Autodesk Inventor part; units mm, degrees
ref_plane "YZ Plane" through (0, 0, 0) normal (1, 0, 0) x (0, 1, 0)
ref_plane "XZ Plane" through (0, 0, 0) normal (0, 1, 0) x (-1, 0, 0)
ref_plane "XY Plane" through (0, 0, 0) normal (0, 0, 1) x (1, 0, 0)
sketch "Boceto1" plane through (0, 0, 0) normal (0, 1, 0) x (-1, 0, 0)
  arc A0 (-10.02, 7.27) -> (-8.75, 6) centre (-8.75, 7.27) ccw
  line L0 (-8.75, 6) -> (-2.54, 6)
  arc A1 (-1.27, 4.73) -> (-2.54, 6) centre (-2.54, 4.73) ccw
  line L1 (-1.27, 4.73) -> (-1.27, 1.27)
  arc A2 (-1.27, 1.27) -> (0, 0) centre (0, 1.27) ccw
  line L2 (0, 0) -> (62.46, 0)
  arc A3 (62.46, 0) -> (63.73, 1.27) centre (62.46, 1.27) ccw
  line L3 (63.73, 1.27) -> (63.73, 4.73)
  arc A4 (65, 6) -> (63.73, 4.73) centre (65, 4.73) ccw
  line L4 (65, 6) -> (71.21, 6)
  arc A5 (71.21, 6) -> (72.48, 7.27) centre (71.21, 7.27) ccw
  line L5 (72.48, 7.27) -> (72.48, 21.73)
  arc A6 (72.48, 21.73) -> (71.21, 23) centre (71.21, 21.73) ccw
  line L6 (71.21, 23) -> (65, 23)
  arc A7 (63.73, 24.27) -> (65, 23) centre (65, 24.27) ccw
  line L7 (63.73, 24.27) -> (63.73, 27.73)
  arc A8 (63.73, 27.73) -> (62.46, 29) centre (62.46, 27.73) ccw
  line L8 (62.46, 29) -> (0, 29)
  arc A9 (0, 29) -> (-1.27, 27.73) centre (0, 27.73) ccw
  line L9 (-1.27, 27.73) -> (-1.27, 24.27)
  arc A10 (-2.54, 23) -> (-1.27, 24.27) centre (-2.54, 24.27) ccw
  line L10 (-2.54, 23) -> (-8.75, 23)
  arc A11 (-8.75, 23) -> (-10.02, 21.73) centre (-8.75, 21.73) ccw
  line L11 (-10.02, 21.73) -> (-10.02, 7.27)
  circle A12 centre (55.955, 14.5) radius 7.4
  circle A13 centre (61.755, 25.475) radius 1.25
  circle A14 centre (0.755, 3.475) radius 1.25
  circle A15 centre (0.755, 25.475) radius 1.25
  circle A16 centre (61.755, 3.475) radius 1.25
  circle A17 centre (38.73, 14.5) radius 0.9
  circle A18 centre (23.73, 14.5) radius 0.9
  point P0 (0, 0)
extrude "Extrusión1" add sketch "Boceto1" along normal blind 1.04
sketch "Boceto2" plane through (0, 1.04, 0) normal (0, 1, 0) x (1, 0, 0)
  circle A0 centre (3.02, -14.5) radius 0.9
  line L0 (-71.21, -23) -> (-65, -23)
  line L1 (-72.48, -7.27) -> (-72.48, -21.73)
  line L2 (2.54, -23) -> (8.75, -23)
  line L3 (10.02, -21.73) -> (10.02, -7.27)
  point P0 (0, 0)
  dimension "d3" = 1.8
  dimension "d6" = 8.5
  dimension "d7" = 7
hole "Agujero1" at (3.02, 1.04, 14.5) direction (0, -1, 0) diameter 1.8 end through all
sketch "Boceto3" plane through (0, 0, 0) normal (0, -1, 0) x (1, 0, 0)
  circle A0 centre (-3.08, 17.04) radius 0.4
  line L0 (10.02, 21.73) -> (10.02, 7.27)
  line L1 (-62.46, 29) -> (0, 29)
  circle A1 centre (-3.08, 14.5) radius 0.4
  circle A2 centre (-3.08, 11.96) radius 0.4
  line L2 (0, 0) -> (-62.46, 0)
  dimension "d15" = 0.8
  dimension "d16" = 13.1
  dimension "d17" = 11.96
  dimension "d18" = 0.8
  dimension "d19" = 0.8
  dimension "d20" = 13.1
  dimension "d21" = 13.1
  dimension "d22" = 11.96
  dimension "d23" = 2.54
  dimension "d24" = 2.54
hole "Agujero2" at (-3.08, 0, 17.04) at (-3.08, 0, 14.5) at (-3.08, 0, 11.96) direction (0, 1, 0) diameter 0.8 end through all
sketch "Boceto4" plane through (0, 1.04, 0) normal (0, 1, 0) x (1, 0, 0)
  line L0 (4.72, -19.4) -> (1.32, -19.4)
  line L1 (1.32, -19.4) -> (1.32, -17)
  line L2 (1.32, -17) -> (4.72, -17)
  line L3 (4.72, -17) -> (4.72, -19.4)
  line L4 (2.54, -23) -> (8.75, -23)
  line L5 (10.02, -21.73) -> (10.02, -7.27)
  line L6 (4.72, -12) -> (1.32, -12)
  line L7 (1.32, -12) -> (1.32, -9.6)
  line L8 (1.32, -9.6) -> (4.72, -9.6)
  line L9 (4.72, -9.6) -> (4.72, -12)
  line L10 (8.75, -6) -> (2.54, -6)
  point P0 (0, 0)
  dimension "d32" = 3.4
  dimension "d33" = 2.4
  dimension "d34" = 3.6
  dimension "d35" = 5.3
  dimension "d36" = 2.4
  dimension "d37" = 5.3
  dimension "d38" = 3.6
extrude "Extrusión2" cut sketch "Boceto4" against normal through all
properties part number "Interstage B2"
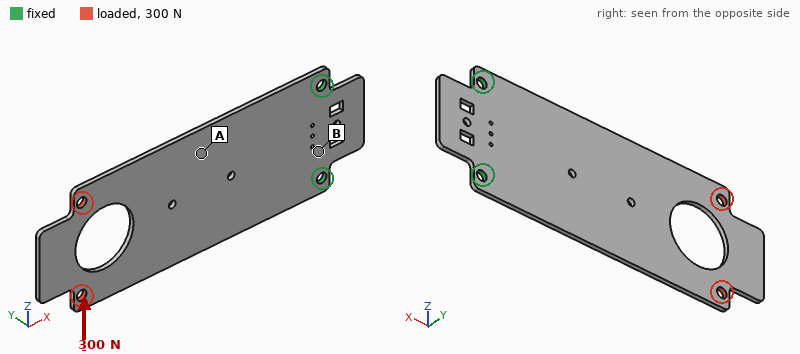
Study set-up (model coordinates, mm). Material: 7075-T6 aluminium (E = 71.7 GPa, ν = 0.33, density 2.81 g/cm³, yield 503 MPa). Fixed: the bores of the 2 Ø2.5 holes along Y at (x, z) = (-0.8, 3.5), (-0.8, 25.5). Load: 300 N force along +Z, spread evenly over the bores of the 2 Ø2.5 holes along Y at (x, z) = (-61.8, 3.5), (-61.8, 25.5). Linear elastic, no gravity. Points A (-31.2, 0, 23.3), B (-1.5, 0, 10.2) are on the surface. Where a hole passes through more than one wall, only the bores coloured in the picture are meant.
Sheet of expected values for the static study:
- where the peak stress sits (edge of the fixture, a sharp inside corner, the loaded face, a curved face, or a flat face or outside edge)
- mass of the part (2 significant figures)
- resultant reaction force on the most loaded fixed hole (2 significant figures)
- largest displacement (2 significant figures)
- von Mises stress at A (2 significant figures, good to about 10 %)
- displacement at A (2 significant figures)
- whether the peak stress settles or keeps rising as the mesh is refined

edge of the fixture
5.7 g
820 N
0.25 mm
40 MPa
0.069 mm
keeps rising
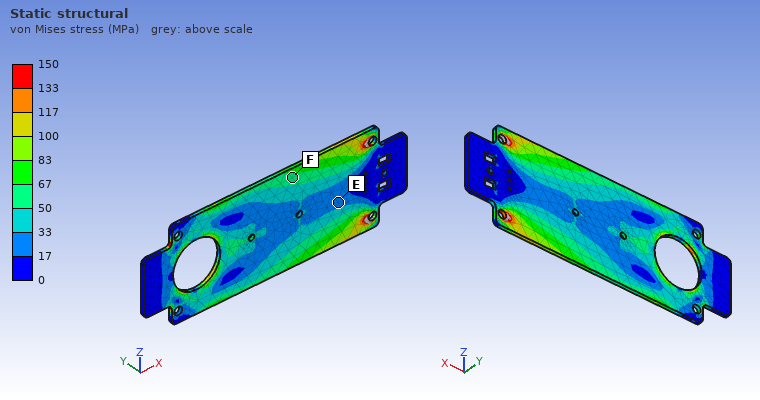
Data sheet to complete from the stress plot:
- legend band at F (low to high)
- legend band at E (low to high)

50 to 67 MPa
17 to 33 MPa
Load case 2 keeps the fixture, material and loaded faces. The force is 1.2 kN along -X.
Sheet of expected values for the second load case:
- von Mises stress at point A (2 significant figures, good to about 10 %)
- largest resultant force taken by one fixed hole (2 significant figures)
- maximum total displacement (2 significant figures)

41 MPa
610 N
57 µm
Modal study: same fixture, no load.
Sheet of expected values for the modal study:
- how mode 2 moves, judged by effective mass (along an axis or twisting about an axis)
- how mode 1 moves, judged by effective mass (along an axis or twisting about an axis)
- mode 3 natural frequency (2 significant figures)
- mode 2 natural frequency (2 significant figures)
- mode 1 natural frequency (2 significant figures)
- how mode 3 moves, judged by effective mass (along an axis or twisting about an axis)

twisting about X
along Y
1000 Hz
980 Hz
200 Hz
along Y
